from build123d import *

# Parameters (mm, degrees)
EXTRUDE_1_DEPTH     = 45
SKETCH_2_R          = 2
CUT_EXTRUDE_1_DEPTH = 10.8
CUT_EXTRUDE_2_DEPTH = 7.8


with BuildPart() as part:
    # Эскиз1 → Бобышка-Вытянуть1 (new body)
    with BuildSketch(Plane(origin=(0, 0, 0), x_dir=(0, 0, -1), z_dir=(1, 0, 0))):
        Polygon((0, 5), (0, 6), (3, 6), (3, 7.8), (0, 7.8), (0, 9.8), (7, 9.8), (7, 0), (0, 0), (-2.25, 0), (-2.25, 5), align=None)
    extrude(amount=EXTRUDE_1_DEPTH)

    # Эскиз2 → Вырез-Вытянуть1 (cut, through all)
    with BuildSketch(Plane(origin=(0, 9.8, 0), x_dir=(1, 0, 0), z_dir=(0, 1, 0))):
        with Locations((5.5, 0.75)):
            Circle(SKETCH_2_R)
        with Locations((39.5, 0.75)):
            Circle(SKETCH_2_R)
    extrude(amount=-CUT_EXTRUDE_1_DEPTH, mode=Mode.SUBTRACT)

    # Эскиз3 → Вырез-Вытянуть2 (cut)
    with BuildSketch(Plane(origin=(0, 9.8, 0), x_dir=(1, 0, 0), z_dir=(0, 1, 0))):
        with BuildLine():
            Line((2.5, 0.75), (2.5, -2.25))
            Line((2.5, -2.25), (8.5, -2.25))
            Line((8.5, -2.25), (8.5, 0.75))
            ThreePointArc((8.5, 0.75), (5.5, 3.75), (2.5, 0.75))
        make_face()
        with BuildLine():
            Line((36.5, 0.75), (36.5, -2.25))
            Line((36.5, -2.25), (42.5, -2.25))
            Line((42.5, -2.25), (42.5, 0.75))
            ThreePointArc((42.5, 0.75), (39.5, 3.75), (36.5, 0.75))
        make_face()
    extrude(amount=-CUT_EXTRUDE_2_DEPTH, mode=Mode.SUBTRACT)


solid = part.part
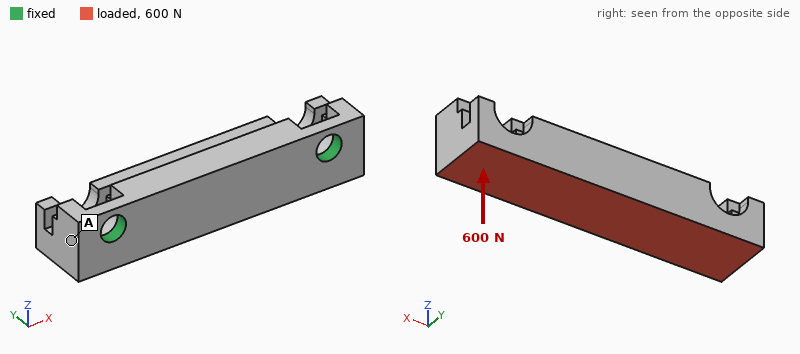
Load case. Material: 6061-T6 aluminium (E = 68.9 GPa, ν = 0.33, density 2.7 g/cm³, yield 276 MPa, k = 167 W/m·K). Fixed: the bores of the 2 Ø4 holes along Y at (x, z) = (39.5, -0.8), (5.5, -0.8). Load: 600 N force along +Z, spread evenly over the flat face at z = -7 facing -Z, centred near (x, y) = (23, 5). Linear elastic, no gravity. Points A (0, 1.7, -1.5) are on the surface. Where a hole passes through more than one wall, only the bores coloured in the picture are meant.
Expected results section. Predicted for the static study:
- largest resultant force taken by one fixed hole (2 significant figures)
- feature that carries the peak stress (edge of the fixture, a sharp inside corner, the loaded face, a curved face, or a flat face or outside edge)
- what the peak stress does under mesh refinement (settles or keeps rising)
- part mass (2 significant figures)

300 N
edge of the fixture
keeps rising
8.1 g
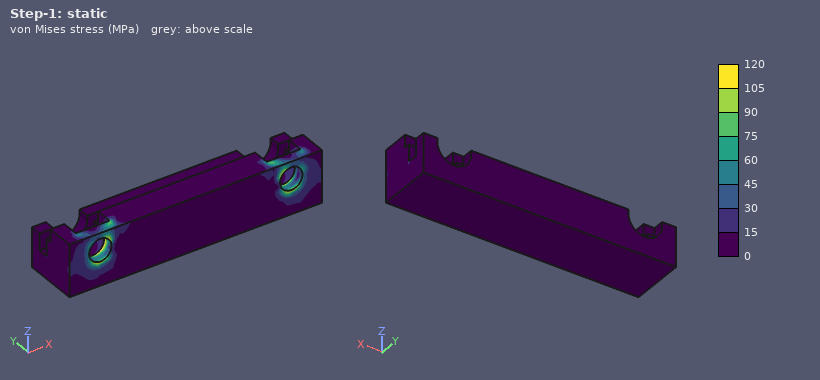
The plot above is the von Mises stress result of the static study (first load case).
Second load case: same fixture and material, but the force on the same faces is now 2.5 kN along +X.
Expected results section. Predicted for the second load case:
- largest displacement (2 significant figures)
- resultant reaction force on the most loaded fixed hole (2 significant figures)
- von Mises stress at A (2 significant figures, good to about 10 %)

14 µm
1.3 kN
14 MPa
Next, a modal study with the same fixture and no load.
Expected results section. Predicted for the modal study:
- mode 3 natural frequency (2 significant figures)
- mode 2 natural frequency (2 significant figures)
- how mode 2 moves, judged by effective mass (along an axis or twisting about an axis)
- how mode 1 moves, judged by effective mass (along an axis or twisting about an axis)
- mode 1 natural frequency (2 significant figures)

23 kHz
21 kHz
along Y
along Z
12 kHz
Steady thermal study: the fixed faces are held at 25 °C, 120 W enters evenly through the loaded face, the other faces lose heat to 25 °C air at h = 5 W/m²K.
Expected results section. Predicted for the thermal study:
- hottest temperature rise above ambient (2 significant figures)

67 K
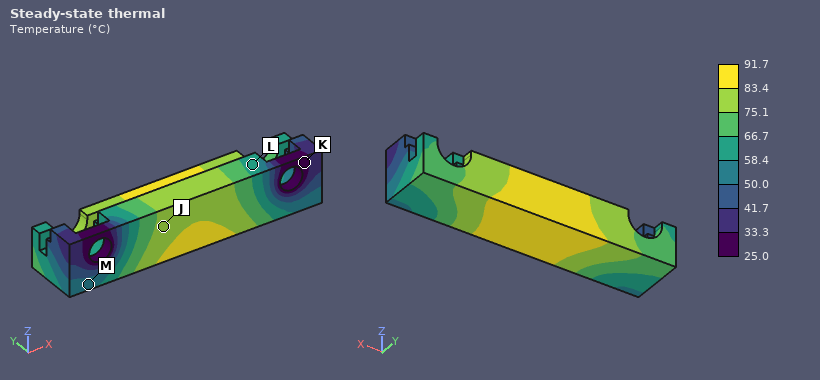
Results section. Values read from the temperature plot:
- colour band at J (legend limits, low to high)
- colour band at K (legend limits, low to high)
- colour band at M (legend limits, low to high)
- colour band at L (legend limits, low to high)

75.1 to 83.4 °C
25.0 to 33.3 °C
50.0 to 58.4 °C
58.4 to 66.7 °C
